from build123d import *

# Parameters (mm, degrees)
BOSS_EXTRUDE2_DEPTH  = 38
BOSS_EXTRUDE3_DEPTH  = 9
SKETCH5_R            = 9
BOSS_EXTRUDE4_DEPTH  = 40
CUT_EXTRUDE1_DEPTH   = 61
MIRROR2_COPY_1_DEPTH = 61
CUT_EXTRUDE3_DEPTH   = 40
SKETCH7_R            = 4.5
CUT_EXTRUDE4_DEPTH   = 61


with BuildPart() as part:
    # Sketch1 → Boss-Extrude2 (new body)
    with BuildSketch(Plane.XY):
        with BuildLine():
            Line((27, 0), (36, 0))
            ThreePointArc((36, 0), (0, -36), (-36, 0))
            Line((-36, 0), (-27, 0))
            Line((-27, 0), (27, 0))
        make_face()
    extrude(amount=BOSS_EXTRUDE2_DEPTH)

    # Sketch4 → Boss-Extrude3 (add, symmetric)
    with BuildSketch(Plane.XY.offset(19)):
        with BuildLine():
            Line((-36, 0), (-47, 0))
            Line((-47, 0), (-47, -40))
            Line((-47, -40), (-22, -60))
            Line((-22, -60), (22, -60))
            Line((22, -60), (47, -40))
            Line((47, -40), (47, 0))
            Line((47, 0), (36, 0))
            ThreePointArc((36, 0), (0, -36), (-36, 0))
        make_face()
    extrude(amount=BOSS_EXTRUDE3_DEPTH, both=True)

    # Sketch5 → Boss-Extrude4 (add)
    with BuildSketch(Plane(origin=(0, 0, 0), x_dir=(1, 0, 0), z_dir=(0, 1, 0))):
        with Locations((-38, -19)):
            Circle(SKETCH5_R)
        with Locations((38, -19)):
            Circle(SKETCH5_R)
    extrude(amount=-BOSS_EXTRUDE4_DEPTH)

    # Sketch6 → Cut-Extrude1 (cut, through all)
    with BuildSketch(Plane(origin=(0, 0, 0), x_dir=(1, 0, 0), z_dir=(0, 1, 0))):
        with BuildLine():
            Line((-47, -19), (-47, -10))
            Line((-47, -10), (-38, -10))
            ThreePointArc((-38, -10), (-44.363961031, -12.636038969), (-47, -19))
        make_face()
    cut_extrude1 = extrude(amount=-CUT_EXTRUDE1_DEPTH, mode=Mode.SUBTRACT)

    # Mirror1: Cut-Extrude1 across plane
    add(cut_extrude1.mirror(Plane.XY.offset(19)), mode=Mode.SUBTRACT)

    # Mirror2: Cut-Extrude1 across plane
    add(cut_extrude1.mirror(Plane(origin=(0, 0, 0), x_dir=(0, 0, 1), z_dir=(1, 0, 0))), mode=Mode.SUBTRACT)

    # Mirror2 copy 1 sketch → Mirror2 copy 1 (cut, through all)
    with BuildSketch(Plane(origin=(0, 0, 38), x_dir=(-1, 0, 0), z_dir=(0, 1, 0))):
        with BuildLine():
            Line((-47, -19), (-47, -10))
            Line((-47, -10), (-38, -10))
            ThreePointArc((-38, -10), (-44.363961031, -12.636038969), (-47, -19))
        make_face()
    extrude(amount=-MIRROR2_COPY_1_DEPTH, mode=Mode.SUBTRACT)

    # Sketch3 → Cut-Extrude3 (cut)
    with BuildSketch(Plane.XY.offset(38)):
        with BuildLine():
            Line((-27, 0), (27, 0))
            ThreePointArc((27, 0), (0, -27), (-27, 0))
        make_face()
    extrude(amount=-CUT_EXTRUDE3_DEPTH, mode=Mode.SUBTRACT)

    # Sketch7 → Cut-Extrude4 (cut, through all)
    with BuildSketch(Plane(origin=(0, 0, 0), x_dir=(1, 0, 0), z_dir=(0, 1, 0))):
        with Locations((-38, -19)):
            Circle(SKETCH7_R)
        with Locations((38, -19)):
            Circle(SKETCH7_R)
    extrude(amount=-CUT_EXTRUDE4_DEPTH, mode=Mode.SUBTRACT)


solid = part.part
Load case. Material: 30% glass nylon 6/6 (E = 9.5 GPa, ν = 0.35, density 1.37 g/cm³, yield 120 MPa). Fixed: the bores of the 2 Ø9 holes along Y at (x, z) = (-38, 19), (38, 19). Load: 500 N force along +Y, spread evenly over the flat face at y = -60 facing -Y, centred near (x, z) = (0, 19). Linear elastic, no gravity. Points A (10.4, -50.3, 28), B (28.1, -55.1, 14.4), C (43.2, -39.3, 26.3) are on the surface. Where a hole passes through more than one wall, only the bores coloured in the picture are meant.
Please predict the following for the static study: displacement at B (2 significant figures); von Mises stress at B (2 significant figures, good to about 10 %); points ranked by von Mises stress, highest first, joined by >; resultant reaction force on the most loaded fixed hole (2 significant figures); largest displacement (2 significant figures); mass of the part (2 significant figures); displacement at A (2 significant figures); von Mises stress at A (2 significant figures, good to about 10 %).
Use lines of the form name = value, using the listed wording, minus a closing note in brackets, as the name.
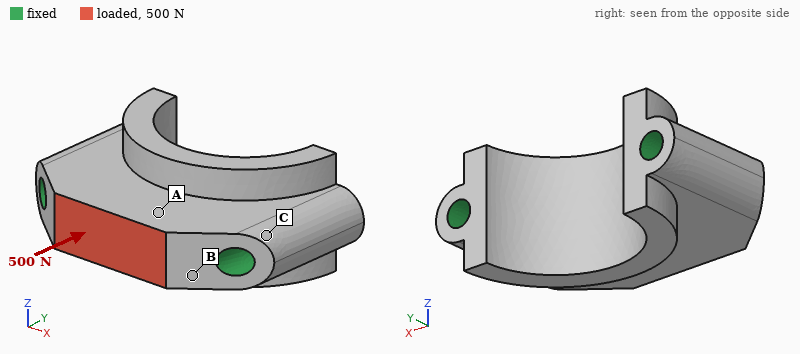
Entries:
displacement at B = 1.2 µm
von Mises stress at B = 0.32 MPa
points ranked by von Mises stress, highest first, joined by > = A > B > C
resultant reaction force on the most loaded fixed hole = 290 N
largest displacement = 3.8 µm
mass of the part = 110 g
displacement at A = 3.0 µm
von Mises stress at A = 0.55 MPa
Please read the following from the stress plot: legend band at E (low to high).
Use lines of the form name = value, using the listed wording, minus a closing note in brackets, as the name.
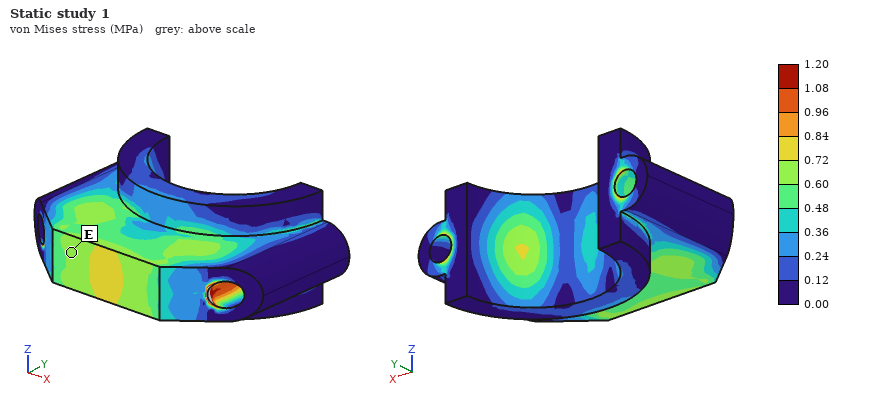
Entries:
legend band at E = 0.60 to 0.72 MPa
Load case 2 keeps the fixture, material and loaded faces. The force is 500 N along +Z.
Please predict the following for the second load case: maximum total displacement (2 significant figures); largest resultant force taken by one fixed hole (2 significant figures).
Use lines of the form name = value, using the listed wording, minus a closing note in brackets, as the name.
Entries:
maximum total displacement = 28 µm
largest resultant force taken by one fixed hole = 250 N
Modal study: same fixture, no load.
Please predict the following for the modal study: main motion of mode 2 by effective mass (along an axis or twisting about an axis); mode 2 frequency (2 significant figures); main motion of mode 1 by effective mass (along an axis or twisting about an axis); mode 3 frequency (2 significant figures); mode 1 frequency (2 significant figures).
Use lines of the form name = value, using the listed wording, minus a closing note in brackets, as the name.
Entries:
main motion of mode 2 by effective mass = along Y
mode 2 frequency = 9600 Hz
main motion of mode 1 by effective mass = along Z
mode 3 frequency = 10 kHz
mode 1 frequency = 5900 Hz
